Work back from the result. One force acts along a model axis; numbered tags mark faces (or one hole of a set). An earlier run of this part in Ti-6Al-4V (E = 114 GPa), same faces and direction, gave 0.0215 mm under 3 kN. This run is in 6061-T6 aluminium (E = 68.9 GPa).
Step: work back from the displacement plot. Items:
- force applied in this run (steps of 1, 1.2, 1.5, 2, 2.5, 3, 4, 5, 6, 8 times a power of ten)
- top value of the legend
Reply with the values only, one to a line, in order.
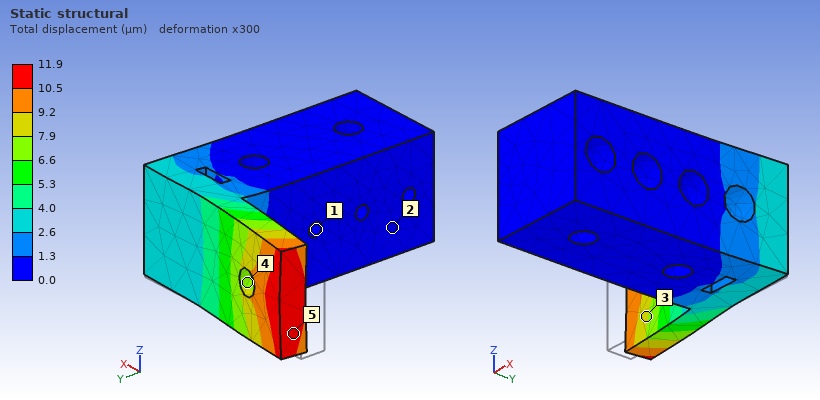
1 kN
11.9 µm
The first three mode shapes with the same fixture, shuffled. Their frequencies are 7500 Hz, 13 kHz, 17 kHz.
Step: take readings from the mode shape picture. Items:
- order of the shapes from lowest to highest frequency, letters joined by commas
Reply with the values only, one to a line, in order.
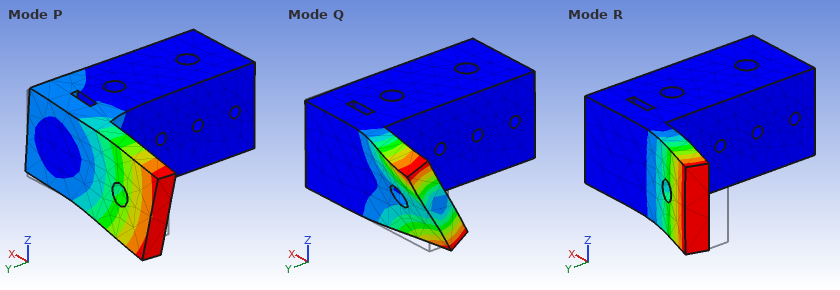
R, P, Q
